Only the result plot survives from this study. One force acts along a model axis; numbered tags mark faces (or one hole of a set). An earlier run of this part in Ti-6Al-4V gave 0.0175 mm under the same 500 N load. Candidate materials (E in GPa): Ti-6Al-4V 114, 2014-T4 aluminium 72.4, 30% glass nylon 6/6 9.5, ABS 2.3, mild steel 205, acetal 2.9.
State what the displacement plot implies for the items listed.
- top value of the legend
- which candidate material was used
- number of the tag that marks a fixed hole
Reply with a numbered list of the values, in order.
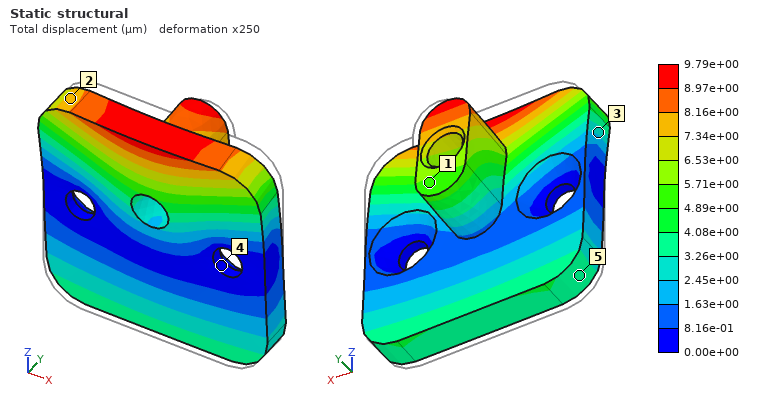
1. 9.79e+00 µm
2. mild steel
3. 4
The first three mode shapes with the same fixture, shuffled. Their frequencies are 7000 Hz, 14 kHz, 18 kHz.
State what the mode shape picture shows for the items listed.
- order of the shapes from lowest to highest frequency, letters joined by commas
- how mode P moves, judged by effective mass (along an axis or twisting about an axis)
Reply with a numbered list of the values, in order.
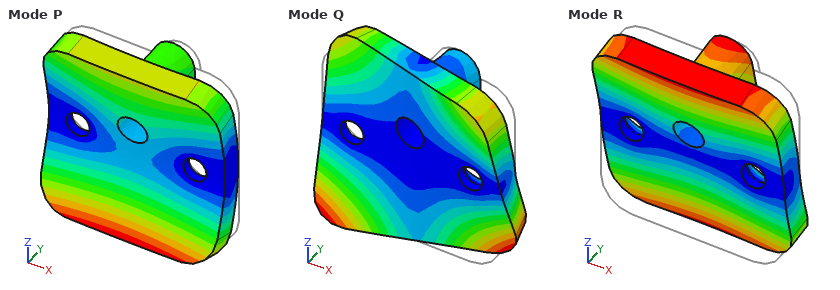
1. R, P, Q
2. along Y
